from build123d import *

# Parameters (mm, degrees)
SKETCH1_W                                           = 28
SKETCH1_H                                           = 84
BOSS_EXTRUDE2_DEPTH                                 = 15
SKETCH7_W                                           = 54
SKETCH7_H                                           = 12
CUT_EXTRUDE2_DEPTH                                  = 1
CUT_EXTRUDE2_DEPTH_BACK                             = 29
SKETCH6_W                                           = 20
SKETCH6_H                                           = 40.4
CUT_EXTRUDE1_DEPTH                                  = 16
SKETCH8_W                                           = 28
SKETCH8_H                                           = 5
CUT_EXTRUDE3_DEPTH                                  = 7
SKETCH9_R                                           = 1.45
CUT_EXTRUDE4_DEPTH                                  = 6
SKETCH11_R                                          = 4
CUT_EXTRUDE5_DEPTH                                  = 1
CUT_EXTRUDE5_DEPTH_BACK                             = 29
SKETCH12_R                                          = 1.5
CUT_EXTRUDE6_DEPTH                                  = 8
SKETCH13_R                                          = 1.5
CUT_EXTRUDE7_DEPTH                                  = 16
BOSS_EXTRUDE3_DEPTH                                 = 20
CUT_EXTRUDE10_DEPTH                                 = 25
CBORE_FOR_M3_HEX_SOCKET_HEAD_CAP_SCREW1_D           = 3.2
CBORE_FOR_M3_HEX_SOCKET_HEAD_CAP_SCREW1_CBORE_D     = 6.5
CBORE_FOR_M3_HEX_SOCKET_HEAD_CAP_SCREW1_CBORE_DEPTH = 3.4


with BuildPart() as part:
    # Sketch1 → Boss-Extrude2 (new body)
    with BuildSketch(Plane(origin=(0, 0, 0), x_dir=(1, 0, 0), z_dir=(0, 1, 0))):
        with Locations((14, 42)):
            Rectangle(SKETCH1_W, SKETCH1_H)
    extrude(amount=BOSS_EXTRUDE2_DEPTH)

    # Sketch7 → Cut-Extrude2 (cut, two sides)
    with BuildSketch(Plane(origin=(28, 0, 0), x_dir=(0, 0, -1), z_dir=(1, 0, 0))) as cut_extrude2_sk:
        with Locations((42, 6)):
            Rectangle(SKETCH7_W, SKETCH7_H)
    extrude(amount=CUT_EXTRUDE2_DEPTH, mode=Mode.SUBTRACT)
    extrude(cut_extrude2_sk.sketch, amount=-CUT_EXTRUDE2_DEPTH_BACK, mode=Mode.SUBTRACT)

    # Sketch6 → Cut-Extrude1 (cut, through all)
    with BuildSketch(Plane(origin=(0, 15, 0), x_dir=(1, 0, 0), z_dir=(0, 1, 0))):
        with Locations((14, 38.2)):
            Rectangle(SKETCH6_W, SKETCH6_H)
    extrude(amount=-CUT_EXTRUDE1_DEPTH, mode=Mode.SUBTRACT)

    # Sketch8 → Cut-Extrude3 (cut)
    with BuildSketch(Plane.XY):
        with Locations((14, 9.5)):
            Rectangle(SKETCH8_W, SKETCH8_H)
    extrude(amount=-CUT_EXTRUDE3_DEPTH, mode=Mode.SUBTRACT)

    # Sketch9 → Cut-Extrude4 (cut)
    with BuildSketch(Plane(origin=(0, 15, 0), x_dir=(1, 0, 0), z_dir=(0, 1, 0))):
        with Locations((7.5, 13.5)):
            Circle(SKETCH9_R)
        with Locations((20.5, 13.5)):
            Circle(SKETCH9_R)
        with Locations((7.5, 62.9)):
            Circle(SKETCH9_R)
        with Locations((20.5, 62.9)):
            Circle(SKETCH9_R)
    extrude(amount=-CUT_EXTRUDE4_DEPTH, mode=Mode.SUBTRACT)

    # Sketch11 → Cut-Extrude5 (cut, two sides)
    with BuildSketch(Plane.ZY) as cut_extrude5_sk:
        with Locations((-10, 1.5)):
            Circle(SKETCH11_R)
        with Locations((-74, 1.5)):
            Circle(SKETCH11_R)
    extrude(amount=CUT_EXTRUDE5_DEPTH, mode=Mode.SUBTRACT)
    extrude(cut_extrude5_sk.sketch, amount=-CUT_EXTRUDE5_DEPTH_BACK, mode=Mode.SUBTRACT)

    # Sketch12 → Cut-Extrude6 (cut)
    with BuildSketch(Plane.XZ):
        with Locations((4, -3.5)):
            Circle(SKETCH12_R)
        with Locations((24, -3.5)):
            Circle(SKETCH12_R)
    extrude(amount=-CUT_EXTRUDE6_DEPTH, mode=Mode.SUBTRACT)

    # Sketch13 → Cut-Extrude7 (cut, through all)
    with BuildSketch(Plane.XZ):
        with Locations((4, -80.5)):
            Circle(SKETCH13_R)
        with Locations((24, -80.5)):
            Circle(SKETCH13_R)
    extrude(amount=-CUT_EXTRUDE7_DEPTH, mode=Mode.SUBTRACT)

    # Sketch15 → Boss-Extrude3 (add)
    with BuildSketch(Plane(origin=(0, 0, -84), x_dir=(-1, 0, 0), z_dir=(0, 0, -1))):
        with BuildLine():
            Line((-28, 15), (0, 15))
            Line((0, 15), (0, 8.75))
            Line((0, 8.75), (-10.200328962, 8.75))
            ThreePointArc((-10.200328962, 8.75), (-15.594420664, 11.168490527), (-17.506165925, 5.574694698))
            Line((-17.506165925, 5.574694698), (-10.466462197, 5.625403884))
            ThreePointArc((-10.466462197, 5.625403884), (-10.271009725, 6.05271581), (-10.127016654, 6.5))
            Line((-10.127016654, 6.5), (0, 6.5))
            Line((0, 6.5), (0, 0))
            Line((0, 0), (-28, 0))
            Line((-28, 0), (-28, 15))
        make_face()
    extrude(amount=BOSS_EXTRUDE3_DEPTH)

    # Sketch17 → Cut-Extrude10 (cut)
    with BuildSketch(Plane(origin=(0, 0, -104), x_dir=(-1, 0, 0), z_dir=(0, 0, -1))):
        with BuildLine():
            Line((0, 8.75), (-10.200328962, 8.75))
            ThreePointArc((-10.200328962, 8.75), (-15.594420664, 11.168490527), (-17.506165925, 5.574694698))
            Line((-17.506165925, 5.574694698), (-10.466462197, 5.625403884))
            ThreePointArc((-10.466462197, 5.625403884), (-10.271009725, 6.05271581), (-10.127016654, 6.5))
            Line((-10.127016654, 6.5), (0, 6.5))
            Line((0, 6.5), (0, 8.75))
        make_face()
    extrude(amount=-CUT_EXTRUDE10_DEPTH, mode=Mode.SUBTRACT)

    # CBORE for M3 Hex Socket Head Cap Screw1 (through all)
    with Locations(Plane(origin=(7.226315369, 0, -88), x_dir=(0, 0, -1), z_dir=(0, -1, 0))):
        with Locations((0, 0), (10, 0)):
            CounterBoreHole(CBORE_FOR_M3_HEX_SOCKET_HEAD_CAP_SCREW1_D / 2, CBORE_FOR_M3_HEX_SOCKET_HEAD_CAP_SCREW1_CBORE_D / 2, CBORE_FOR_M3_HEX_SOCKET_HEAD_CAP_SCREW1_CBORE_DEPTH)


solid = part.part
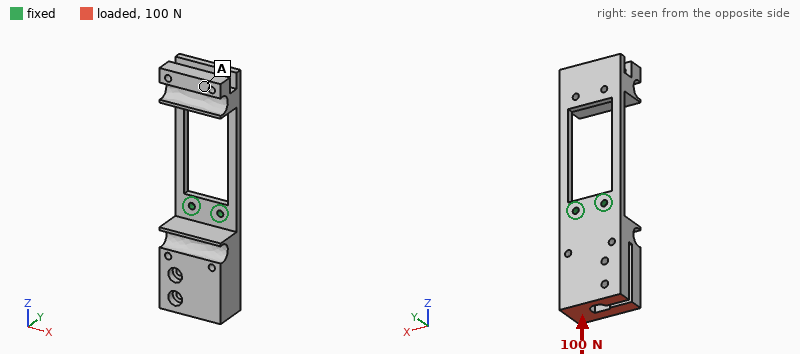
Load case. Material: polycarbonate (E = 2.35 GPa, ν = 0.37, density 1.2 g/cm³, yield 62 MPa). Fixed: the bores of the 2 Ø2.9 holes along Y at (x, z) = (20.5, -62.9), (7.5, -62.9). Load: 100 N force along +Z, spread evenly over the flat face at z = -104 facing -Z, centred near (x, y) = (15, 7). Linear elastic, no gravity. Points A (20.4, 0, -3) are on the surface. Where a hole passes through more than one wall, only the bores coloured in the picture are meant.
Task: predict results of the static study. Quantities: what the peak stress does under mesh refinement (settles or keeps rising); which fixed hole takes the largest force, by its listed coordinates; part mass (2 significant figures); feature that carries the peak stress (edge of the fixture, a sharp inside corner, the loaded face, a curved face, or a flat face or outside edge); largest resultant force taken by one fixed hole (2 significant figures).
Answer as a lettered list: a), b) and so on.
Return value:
a) keeps rising
b) (20.5, -62.9)
c) 21 g
d) edge of the fixture
e) 54 N
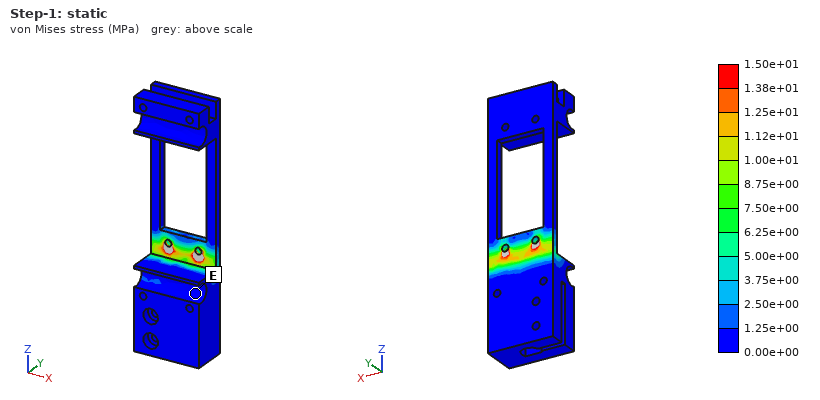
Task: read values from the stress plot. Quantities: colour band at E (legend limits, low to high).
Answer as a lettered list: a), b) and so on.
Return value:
a) 0.00e+00 to 1.25e+00 MPa
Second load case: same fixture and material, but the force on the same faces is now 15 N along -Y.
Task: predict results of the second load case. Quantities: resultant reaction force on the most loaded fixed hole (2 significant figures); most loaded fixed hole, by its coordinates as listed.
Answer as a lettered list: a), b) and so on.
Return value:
a) 8.0 N
b) (20.5, -62.9)
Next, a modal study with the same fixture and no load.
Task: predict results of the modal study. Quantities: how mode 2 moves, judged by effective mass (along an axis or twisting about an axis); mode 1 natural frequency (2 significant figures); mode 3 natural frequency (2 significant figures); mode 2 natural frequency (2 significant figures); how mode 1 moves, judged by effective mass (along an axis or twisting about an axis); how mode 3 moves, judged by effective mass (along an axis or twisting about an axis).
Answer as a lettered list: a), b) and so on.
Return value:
a) along X
b) 61 Hz
c) 260 Hz
d) 180 Hz
e) along Y
f) along Y
